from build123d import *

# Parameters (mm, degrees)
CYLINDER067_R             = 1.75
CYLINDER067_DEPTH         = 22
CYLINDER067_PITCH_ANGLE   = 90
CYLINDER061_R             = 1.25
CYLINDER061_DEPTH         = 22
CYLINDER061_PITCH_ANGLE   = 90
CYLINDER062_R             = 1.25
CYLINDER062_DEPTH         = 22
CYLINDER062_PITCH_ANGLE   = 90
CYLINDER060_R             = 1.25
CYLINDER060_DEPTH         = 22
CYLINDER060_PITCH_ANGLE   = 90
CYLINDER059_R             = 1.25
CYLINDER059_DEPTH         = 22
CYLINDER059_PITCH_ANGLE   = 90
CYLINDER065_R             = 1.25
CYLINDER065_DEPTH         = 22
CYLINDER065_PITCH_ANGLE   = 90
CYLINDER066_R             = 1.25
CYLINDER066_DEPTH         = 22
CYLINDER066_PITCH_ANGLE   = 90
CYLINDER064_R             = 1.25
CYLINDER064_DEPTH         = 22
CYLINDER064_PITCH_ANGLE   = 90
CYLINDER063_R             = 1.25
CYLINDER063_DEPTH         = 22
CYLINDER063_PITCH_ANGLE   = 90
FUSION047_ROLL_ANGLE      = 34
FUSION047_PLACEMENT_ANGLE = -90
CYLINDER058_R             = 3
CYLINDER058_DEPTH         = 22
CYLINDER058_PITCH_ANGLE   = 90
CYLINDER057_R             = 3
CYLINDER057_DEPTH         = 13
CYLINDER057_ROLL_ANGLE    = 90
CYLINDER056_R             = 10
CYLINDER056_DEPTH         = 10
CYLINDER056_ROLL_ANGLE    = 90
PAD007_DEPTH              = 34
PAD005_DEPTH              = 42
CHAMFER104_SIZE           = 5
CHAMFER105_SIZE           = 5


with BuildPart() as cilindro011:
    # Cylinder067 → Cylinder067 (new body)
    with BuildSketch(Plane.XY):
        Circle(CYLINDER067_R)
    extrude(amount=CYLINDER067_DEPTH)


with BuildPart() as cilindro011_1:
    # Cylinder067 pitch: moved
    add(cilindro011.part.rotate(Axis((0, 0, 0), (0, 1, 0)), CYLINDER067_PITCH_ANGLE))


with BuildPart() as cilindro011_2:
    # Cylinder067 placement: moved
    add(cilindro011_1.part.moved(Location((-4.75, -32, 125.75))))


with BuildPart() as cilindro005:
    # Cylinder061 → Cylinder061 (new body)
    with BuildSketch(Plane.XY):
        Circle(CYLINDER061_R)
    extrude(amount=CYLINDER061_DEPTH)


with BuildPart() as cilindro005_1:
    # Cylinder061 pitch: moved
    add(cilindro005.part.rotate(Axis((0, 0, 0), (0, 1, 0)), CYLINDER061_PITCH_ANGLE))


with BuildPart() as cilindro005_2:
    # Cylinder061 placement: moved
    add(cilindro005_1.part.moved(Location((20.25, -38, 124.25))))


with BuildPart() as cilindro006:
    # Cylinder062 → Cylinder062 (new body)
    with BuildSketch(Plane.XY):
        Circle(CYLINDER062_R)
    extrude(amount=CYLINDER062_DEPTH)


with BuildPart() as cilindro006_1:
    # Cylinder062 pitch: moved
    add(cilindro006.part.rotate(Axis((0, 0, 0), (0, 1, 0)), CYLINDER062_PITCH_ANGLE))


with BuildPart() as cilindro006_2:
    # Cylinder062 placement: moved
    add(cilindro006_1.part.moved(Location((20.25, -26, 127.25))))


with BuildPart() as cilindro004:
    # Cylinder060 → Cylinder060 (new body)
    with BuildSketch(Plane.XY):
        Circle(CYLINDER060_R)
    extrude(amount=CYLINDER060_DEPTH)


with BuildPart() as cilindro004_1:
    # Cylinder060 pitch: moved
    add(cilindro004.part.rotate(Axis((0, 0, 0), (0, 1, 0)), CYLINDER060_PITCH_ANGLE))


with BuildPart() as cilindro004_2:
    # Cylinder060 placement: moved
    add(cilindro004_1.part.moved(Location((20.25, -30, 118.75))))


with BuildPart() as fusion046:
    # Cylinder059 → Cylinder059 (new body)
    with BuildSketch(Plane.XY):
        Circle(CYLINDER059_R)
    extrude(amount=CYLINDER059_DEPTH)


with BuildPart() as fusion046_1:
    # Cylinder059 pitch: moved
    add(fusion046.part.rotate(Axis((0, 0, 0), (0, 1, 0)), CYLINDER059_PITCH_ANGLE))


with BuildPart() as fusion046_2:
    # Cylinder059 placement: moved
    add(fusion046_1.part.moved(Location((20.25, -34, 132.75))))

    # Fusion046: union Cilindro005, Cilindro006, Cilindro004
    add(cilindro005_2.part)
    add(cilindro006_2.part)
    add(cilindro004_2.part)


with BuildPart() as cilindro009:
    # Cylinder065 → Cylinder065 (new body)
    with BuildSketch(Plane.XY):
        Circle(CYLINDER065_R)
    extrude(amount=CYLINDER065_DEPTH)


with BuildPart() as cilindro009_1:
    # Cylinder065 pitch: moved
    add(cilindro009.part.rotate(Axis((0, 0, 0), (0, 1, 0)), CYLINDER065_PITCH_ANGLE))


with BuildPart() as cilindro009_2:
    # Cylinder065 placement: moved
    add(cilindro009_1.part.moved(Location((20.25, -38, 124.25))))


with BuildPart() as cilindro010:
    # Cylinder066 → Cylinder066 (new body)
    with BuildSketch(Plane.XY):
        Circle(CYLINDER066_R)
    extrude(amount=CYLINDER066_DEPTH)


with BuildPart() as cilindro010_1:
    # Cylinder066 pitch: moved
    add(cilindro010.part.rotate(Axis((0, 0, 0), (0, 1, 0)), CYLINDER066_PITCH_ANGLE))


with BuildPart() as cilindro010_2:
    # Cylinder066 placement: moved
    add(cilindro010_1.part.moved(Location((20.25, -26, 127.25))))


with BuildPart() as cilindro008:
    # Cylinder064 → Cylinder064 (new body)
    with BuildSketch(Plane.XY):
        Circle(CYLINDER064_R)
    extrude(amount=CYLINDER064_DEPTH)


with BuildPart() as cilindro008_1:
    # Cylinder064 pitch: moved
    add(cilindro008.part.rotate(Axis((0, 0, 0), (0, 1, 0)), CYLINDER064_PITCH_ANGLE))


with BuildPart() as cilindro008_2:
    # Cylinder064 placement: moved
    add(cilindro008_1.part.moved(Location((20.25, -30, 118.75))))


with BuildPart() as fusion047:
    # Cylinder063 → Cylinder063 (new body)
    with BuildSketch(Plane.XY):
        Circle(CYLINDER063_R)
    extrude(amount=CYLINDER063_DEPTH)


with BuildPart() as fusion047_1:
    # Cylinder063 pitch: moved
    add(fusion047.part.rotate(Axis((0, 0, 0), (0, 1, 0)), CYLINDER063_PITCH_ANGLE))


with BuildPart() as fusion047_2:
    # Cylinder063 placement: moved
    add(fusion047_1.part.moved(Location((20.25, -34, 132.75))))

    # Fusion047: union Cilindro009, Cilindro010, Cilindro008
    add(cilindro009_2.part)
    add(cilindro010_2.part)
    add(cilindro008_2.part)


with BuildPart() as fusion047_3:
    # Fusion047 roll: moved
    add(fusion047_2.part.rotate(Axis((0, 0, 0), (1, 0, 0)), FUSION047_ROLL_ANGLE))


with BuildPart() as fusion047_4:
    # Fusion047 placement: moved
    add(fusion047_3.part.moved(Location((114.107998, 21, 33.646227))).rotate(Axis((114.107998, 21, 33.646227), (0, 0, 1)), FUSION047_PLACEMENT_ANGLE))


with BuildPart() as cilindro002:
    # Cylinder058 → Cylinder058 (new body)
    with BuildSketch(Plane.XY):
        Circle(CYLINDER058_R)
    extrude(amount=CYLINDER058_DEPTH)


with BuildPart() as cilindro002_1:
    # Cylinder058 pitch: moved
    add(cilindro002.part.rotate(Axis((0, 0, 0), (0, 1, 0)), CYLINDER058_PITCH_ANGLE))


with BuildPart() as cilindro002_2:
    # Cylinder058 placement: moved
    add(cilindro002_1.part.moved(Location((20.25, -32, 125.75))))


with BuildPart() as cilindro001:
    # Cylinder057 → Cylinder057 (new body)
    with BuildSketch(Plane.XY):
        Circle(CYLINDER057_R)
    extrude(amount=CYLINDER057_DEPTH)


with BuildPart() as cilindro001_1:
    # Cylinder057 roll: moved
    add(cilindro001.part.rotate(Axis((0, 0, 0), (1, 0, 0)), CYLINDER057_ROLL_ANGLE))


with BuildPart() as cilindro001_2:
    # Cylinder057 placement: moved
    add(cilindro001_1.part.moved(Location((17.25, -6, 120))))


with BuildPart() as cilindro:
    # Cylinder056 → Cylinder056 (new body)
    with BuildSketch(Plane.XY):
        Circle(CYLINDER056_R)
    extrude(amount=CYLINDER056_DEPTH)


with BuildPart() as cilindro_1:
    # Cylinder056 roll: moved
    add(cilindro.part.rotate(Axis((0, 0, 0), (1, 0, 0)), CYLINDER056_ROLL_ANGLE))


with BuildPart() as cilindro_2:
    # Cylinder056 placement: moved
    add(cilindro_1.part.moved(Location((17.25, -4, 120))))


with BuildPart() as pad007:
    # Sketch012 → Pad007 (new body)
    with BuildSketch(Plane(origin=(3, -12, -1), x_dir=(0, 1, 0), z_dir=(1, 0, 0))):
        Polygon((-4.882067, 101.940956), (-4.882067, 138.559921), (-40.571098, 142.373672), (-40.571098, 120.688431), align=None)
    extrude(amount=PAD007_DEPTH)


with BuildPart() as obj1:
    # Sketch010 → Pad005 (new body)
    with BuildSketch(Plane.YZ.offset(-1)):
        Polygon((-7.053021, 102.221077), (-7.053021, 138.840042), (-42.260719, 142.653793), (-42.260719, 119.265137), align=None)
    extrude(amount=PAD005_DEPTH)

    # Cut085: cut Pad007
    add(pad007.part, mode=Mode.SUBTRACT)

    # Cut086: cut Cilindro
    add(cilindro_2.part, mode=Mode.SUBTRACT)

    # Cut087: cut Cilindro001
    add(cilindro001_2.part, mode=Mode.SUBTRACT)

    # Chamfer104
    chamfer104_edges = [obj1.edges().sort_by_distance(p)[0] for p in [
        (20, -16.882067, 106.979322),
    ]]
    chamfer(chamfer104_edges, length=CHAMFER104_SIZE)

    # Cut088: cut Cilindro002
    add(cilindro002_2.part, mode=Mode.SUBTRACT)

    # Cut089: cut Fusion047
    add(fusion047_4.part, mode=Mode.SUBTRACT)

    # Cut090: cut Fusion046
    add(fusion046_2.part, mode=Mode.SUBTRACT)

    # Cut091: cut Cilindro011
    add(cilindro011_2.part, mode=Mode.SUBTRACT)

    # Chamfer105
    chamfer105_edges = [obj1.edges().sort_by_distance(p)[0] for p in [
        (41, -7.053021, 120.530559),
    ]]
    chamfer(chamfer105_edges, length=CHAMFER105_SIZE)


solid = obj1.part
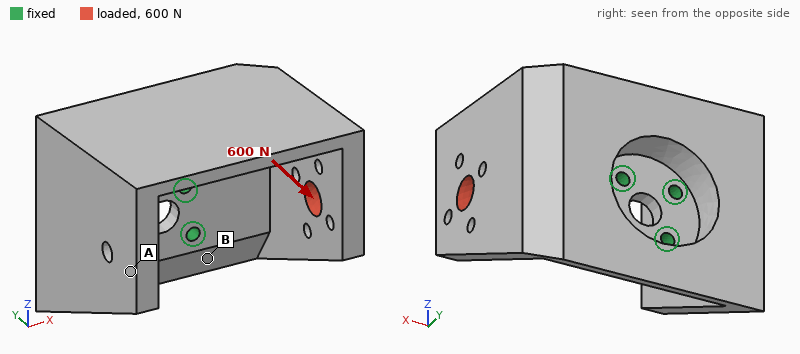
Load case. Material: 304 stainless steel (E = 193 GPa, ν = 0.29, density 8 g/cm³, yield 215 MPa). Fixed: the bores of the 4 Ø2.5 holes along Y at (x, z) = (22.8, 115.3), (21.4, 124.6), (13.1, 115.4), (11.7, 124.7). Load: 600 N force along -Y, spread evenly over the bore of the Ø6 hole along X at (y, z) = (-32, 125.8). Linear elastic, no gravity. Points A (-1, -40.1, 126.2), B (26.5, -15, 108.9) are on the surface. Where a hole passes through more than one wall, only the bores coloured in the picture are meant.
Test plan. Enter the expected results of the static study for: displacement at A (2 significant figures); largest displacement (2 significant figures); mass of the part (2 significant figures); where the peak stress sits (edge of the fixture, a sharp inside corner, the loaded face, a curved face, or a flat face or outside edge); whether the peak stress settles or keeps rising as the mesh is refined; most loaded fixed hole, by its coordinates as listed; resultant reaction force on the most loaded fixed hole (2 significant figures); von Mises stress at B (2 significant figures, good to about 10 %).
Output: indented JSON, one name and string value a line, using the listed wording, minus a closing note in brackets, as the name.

{
  "displacement at A": "14 µm",
  "largest displacement": "25 µm",
  "mass of the part": "150 g",
  "where the peak stress sits": "edge of the fixture",
  "whether the peak stress settles or keeps rising as the mesh is refined": "keeps rising",
  "most loaded fixed hole, by its coordinates as listed": "(21.4, 124.6)",
  "resultant reaction force on the most loaded fixed hole": "780 N",
  "von Mises stress at B": "17 MPa"
}
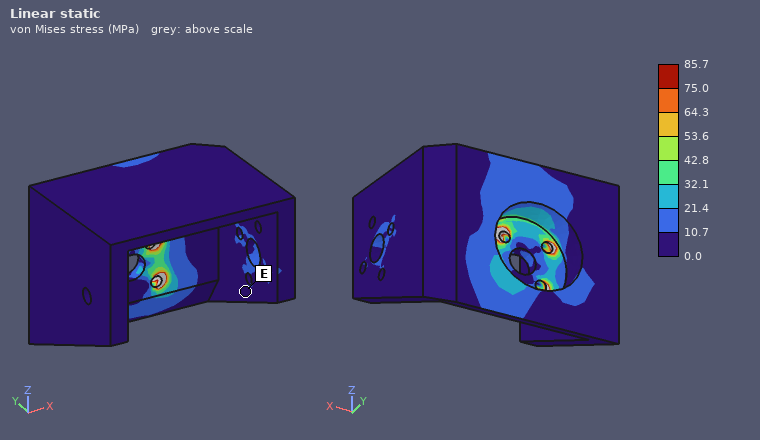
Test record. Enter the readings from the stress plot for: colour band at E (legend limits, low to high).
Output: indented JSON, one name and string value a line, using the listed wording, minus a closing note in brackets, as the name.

{
  "colour band at E": "0.0 to 10.7 MPa"
}
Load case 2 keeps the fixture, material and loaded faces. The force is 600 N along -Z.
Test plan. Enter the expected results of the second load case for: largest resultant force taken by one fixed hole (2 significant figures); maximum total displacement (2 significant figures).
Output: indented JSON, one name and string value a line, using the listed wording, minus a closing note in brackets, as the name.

{
  "largest resultant force taken by one fixed hole": "750 N",
  "maximum total displacement": "29 µm"
}
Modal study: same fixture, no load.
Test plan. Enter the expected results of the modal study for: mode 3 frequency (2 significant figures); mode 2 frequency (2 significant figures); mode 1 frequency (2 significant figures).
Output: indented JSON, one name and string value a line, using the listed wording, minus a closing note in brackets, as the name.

{
  "mode 3 frequency": "6800 Hz",
  "mode 2 frequency": "4400 Hz",
  "mode 1 frequency": "3400 Hz"
}
